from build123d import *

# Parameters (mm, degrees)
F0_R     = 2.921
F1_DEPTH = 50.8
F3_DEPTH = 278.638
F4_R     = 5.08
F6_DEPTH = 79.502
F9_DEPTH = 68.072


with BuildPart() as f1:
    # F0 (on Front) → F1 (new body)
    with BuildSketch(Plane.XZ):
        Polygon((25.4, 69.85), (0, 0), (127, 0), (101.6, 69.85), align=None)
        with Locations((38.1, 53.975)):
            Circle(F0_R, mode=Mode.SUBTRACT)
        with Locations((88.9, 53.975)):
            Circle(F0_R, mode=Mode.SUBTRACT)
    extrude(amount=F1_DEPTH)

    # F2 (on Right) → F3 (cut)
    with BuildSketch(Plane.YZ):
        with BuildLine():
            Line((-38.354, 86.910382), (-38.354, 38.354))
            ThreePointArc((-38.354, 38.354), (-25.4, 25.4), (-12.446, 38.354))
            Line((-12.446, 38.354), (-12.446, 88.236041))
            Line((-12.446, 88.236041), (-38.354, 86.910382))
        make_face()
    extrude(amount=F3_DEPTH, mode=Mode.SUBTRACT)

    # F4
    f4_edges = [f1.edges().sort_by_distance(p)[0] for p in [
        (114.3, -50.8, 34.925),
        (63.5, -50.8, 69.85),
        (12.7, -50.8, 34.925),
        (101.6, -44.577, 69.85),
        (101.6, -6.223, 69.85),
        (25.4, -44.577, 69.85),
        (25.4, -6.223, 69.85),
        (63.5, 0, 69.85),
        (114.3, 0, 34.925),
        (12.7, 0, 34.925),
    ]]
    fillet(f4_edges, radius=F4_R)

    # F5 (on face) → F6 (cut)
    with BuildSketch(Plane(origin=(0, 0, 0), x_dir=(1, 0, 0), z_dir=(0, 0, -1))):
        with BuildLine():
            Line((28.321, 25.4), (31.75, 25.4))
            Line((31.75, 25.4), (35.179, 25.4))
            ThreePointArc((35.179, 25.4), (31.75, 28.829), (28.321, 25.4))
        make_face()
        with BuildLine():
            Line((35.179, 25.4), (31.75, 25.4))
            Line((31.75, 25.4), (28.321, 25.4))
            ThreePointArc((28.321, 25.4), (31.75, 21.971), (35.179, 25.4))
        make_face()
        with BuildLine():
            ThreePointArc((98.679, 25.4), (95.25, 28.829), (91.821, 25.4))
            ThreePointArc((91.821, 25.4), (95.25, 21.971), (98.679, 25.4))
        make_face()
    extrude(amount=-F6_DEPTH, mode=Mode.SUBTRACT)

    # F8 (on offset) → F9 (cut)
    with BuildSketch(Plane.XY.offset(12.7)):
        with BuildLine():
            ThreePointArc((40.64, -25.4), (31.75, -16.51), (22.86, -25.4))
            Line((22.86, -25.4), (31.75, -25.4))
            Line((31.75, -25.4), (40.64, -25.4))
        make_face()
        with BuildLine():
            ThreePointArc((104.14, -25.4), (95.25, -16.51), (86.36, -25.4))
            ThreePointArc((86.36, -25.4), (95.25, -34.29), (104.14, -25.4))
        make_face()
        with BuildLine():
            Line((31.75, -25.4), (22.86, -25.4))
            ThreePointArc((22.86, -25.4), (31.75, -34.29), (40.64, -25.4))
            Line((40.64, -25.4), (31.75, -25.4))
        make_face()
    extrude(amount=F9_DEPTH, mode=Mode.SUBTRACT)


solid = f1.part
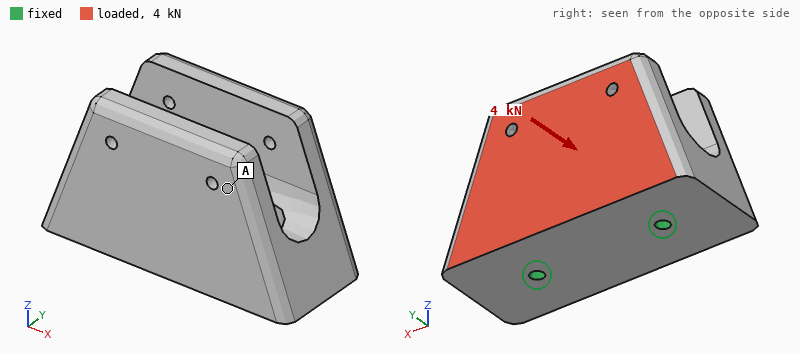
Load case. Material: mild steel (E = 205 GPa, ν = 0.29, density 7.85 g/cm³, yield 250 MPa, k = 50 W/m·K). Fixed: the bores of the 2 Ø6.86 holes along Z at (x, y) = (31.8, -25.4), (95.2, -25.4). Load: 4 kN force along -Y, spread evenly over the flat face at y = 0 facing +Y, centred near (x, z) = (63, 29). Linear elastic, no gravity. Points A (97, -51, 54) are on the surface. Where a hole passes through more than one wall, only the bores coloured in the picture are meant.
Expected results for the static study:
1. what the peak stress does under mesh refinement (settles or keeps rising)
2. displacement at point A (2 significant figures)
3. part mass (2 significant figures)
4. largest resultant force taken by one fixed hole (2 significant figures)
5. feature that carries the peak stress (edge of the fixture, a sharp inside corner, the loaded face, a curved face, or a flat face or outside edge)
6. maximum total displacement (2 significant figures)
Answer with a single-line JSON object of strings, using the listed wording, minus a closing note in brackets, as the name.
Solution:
{"what the peak stress does under mesh refinement": "keeps rising", "displacement at point A": "13 µm", "part mass": "2.0 kg", "largest resultant force taken by one fixed hole": "2.0 kN", "feature that carries the peak stress": "edge of the fixture", "maximum total displacement": "24 µm"}
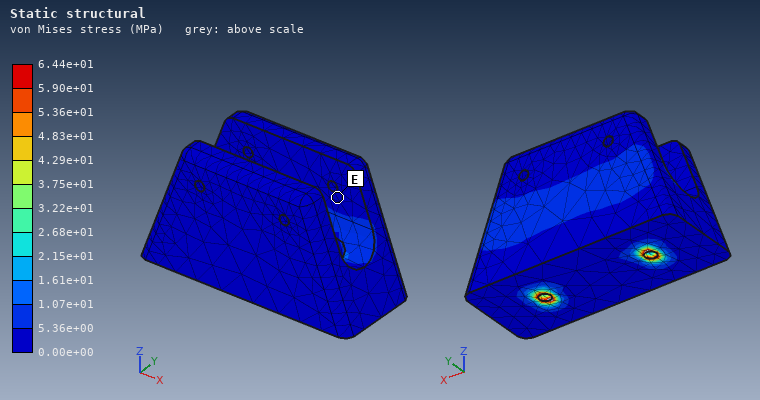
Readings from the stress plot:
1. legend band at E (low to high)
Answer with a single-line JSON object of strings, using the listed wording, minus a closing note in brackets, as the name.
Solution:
{"legend band at E": "0.00e+00 to 5.36e+00 MPa"}
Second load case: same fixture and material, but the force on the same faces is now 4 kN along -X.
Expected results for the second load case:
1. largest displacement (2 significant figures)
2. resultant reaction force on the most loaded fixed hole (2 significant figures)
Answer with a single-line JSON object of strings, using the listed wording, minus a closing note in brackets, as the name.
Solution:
{"largest displacement": "2.8 µm", "resultant reaction force on the most loaded fixed hole": "2.8 kN"}
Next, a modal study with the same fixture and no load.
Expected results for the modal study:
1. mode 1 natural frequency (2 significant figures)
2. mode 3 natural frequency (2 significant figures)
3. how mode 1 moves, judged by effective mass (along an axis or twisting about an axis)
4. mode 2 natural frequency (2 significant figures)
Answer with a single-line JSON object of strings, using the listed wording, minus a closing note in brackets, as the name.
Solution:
{"mode 1 natural frequency": "2100 Hz", "mode 3 natural frequency": "5600 Hz", "how mode 1 moves, judged by effective mass": "along Y", "mode 2 natural frequency": "5000 Hz"}
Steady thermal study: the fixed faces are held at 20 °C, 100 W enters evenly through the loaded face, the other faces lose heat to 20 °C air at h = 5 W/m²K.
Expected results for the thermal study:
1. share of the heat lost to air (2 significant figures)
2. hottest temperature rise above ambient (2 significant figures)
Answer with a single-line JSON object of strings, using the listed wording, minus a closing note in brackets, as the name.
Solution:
{"share of the heat lost to air": "3.6 %", "hottest temperature rise above ambient": "49 K"}
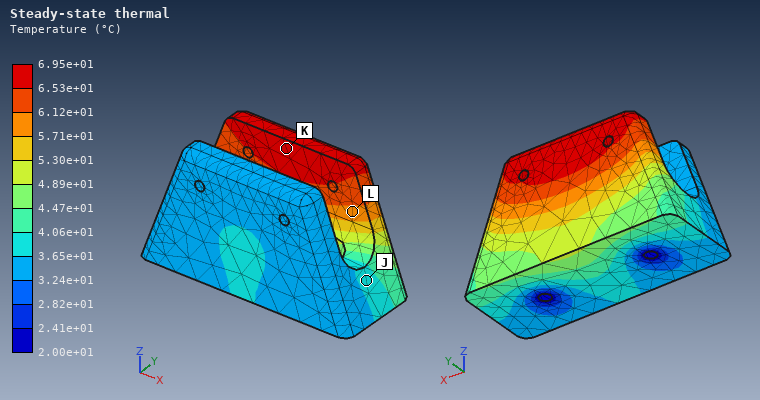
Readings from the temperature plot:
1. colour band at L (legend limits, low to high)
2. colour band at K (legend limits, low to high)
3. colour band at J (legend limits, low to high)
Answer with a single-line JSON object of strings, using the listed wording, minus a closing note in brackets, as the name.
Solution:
{"colour band at L": "5.71e+01 to 6.12e+01 °C", "colour band at K": "6.53e+01 to 6.95e+01 °C", "colour band at J": "3.65e+01 to 4.06e+01 °C"}
